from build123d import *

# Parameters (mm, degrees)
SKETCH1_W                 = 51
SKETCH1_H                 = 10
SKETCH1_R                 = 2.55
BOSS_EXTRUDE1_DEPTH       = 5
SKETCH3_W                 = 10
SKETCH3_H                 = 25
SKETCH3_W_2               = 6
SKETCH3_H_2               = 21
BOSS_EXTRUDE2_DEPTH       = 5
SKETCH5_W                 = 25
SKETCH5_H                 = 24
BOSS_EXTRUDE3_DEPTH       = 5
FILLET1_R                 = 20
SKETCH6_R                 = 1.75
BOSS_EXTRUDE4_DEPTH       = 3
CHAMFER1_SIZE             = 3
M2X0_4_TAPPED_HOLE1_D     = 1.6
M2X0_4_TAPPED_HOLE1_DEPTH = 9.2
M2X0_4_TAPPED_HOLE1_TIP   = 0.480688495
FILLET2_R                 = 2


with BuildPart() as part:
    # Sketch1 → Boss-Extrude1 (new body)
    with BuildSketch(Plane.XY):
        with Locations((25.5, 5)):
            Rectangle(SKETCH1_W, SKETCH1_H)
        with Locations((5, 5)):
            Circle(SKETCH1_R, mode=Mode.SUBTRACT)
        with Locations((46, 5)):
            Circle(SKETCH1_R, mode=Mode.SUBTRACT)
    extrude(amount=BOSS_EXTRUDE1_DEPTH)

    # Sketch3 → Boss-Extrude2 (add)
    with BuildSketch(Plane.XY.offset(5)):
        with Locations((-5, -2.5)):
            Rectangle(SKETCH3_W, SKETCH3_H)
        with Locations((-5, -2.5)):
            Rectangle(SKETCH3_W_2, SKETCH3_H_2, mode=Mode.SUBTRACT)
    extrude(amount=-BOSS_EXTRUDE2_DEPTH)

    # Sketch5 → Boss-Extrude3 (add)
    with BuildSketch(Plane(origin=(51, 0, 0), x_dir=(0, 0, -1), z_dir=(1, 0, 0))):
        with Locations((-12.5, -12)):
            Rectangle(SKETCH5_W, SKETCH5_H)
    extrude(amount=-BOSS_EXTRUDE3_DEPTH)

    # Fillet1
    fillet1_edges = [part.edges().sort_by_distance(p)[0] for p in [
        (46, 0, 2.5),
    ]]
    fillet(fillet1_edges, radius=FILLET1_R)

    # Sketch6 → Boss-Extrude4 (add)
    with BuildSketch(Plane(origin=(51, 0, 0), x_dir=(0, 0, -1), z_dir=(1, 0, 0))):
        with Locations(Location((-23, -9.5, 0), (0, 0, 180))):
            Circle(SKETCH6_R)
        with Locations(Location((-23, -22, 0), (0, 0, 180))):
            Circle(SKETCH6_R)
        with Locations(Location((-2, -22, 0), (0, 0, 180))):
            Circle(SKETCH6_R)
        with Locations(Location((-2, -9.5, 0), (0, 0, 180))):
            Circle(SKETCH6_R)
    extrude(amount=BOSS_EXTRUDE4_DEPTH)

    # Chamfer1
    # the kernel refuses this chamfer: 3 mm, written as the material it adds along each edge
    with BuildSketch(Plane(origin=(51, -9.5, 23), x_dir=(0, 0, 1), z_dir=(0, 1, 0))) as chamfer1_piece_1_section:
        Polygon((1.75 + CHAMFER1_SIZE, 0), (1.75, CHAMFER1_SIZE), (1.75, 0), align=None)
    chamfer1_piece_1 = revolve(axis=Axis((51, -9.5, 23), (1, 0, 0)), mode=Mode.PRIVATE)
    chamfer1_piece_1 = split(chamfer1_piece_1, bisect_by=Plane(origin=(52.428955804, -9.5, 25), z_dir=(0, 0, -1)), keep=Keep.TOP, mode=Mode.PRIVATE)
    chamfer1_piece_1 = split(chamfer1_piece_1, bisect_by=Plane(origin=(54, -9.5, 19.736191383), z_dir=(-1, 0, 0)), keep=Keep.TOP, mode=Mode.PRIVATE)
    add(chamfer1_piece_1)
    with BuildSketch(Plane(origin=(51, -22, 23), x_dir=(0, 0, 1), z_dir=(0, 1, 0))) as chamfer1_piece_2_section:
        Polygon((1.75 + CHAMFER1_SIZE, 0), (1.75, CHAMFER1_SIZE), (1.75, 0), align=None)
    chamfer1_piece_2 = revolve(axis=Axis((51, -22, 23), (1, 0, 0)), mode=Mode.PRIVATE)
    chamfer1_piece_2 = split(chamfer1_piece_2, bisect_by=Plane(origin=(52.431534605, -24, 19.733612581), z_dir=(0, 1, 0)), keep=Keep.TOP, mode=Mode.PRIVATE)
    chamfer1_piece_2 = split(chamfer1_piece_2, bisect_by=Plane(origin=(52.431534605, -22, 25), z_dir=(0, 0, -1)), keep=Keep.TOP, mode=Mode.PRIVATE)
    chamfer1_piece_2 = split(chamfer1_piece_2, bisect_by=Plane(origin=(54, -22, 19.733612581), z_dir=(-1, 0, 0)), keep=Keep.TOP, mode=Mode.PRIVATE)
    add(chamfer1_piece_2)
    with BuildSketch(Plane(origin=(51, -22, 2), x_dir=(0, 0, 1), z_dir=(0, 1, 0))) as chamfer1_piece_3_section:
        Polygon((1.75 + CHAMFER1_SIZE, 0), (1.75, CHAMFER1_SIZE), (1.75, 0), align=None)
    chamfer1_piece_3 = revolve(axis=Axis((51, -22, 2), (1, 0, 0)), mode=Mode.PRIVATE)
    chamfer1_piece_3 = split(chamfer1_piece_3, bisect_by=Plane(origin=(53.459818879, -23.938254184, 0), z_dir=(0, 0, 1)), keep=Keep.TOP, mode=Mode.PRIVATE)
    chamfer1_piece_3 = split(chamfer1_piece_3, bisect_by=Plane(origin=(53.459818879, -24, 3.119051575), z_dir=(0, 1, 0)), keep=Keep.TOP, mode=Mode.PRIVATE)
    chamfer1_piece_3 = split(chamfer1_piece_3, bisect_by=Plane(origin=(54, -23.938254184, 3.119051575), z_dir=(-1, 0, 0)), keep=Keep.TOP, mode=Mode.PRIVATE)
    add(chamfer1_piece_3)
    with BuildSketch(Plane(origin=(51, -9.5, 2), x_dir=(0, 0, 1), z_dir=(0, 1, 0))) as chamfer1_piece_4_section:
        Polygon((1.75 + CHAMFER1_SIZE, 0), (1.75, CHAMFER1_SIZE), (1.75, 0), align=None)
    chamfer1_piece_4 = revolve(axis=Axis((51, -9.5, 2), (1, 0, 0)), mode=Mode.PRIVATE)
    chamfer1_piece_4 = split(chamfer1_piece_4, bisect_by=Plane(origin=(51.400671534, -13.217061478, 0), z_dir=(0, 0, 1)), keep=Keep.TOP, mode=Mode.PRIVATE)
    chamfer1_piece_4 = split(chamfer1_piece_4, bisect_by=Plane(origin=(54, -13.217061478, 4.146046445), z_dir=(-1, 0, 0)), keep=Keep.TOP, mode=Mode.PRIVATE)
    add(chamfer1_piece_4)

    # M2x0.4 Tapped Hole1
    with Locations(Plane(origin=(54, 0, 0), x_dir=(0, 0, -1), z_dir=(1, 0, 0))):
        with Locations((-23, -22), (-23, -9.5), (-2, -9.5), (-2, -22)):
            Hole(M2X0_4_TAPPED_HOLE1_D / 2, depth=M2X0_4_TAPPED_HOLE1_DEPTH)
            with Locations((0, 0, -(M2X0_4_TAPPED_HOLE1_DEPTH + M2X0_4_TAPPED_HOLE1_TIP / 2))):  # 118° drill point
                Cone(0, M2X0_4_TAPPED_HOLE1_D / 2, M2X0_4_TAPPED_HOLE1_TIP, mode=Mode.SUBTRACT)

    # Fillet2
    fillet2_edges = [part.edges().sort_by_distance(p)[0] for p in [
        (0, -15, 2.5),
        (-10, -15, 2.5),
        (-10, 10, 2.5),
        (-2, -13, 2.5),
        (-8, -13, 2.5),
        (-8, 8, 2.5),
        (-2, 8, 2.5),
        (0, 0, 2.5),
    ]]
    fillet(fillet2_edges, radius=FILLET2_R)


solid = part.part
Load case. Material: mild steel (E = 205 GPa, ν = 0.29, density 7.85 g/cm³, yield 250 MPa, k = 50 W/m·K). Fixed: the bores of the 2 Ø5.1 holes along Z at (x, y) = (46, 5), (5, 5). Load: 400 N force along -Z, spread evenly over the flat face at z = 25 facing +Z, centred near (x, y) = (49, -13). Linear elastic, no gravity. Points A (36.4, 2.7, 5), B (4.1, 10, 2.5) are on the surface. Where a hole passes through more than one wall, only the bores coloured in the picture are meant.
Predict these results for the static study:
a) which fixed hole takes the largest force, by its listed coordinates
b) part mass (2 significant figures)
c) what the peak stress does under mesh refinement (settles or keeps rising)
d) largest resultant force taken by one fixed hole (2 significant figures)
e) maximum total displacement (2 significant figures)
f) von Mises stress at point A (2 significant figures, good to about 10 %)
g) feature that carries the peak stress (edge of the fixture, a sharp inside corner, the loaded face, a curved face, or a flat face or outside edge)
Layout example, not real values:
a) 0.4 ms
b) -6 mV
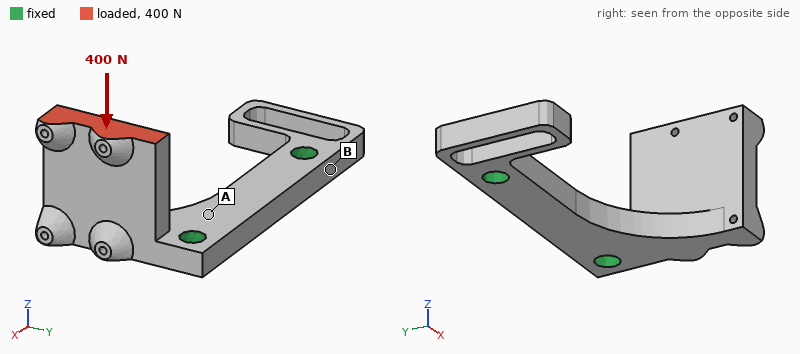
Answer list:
a) (46, 5)
b) 52 g
c) keeps rising
d) 420 N
e) 52 µm
f) 20 MPa
g) edge of the fixture
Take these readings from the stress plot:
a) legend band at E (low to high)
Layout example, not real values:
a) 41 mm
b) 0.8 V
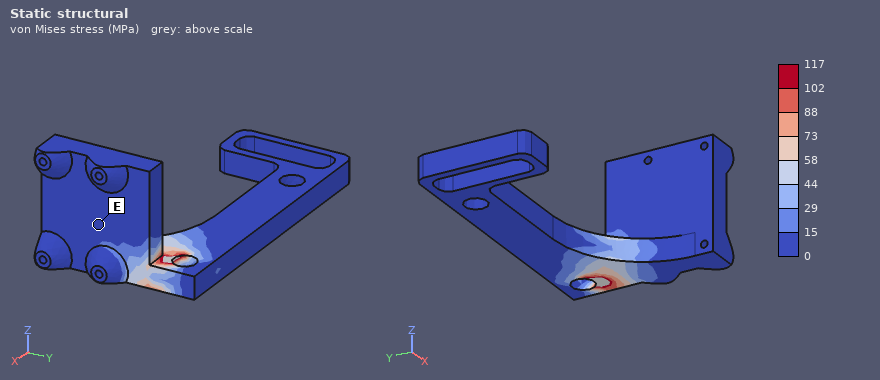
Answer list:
a) 0 to 15 MPa
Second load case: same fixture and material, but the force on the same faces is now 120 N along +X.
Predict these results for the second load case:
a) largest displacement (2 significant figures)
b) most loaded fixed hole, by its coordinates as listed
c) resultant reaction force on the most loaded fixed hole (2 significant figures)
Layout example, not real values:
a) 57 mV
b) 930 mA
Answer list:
a) 31 µm
b) (46, 5)
c) 94 N
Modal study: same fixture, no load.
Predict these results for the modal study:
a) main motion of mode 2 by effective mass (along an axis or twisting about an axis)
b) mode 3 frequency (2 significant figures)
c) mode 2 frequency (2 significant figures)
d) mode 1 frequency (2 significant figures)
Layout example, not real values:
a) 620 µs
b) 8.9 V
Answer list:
a) along X
b) 5000 Hz
c) 3900 Hz
d) 3000 Hz
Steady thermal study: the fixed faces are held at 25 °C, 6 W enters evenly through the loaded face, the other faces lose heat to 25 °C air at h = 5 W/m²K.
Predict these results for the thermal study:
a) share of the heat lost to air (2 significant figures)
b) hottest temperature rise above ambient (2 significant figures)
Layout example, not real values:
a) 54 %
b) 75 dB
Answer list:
a) 4.6 %
b) 42 K
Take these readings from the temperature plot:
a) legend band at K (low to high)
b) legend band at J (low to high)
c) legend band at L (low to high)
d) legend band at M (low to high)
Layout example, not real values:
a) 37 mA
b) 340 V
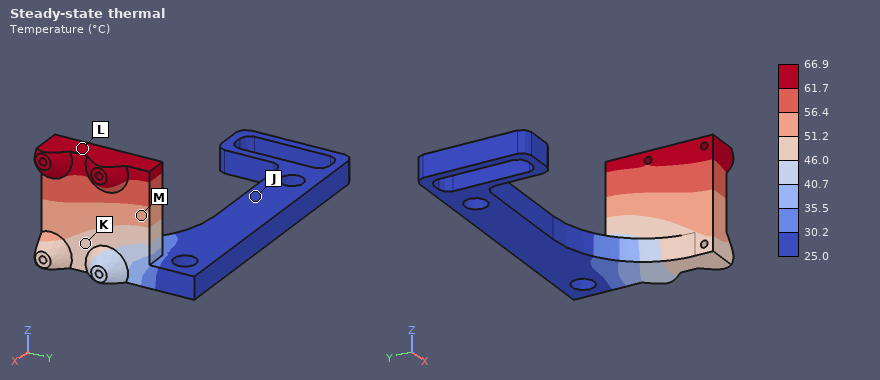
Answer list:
a) 46.0 to 51.2 °C
b) 25.0 to 30.2 °C
c) 61.7 to 66.9 °C
d) 51.2 to 56.4 °C
